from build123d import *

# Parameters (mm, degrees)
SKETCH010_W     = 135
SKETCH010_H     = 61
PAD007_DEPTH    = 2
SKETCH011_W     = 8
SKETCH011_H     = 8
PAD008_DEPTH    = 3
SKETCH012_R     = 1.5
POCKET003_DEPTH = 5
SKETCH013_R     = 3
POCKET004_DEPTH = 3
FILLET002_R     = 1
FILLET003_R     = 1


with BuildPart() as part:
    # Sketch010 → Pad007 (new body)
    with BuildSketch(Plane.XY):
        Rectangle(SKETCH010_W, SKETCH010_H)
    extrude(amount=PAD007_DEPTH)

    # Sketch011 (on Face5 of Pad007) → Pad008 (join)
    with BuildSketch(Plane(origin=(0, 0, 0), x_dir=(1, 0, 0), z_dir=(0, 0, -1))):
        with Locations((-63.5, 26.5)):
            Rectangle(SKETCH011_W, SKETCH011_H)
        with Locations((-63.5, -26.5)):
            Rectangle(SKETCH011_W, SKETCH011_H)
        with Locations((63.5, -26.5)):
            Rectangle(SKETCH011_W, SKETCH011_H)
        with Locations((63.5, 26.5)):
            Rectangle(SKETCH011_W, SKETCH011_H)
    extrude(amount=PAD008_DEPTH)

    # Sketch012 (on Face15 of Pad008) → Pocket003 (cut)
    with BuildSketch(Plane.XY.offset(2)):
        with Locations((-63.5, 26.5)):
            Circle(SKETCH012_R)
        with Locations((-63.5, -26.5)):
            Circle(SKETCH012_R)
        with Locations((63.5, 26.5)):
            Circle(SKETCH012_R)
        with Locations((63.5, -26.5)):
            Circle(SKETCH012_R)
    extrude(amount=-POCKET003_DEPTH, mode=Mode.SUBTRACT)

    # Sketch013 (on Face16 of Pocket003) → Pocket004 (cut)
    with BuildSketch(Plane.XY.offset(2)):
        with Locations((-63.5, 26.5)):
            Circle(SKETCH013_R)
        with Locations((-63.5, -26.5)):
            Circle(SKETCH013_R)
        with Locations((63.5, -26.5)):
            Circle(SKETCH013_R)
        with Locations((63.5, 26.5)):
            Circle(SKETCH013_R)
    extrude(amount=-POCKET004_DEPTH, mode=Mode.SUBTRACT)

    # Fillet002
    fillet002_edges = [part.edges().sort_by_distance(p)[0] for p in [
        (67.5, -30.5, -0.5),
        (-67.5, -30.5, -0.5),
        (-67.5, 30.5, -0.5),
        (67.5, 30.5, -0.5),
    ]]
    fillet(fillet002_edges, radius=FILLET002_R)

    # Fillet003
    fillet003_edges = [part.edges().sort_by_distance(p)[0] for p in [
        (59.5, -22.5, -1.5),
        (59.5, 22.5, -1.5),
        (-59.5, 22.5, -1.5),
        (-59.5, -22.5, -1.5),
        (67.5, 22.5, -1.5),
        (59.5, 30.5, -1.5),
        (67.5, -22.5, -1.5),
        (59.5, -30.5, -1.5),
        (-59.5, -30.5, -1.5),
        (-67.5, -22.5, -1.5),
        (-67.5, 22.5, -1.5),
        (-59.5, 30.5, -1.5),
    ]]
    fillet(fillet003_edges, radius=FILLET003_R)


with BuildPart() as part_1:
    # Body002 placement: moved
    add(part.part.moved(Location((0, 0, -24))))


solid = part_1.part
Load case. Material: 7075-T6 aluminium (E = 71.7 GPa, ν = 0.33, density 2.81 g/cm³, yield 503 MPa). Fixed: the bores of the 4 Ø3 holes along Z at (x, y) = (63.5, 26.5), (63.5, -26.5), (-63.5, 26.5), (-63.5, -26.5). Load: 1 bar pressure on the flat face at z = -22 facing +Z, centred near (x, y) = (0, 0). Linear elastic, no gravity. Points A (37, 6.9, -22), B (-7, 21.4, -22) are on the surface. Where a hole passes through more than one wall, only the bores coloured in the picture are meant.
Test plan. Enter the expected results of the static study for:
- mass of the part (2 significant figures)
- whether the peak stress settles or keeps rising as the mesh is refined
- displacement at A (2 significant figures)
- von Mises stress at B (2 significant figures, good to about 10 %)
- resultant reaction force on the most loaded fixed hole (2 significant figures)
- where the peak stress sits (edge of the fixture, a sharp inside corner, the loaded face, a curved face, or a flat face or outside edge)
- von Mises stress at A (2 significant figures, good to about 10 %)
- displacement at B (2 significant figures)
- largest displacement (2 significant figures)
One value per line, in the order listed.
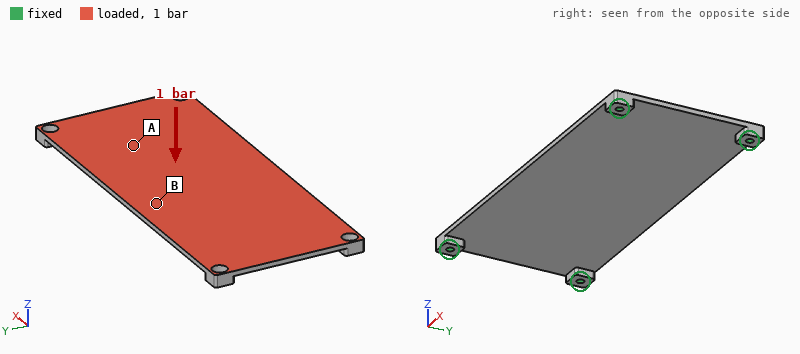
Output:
47 g
keeps rising
0.81 mm
110 MPa
630 N
a sharp inside corner
28 MPa
1.6 mm
1.7 mm
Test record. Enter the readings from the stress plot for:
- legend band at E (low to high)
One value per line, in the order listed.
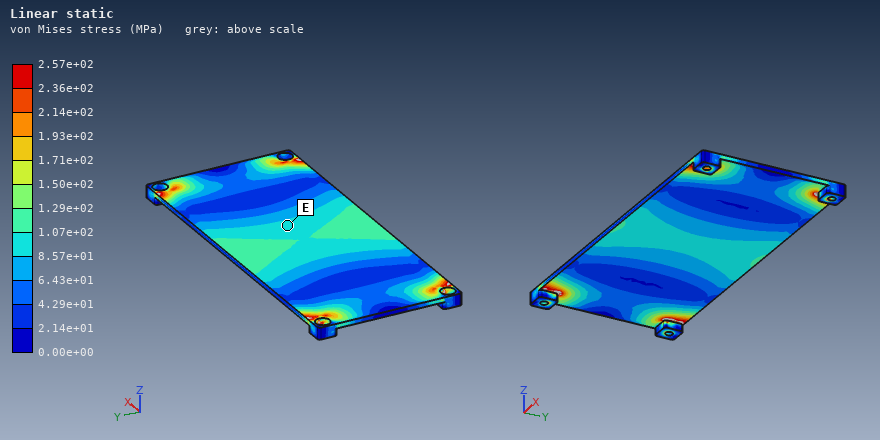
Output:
8.57e+01 to 1.07e+02 MPa
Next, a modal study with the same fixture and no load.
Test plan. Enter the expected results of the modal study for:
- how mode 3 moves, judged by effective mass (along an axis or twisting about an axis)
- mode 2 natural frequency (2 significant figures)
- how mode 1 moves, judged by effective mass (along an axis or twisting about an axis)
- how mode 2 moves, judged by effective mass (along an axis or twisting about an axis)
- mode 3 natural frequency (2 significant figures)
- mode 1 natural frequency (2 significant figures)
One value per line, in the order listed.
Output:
twisting about Y
1100 Hz
along Z
twisting about X
1600 Hz
600 Hz
